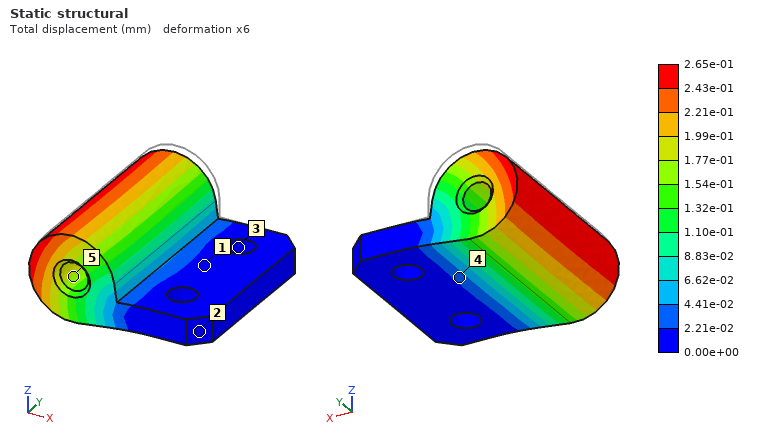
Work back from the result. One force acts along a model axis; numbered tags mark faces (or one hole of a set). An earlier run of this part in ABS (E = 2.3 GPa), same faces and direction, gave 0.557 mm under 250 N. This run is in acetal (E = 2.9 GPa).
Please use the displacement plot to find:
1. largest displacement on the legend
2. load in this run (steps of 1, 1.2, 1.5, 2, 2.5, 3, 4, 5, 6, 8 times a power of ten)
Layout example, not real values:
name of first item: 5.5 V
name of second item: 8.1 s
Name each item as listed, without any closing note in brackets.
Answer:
largest displacement on the legend: 2.65e-01 mm
load in this run: 150 N
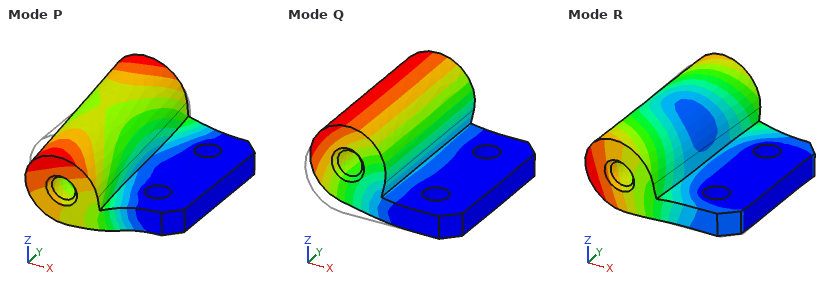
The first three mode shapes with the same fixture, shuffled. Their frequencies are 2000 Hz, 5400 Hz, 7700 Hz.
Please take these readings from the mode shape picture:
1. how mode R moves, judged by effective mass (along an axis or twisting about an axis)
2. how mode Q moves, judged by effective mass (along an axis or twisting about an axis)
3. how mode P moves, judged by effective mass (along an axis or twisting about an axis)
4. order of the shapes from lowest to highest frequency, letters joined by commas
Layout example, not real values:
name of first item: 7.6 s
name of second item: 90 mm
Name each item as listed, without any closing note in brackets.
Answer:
how mode R moves, judged by effective mass: along Y
how mode Q moves, judged by effective mass: along Z
how mode P moves, judged by effective mass: along Y
order of the shapes from lowest to highest frequency, letters joined by commas: Q, P, R
